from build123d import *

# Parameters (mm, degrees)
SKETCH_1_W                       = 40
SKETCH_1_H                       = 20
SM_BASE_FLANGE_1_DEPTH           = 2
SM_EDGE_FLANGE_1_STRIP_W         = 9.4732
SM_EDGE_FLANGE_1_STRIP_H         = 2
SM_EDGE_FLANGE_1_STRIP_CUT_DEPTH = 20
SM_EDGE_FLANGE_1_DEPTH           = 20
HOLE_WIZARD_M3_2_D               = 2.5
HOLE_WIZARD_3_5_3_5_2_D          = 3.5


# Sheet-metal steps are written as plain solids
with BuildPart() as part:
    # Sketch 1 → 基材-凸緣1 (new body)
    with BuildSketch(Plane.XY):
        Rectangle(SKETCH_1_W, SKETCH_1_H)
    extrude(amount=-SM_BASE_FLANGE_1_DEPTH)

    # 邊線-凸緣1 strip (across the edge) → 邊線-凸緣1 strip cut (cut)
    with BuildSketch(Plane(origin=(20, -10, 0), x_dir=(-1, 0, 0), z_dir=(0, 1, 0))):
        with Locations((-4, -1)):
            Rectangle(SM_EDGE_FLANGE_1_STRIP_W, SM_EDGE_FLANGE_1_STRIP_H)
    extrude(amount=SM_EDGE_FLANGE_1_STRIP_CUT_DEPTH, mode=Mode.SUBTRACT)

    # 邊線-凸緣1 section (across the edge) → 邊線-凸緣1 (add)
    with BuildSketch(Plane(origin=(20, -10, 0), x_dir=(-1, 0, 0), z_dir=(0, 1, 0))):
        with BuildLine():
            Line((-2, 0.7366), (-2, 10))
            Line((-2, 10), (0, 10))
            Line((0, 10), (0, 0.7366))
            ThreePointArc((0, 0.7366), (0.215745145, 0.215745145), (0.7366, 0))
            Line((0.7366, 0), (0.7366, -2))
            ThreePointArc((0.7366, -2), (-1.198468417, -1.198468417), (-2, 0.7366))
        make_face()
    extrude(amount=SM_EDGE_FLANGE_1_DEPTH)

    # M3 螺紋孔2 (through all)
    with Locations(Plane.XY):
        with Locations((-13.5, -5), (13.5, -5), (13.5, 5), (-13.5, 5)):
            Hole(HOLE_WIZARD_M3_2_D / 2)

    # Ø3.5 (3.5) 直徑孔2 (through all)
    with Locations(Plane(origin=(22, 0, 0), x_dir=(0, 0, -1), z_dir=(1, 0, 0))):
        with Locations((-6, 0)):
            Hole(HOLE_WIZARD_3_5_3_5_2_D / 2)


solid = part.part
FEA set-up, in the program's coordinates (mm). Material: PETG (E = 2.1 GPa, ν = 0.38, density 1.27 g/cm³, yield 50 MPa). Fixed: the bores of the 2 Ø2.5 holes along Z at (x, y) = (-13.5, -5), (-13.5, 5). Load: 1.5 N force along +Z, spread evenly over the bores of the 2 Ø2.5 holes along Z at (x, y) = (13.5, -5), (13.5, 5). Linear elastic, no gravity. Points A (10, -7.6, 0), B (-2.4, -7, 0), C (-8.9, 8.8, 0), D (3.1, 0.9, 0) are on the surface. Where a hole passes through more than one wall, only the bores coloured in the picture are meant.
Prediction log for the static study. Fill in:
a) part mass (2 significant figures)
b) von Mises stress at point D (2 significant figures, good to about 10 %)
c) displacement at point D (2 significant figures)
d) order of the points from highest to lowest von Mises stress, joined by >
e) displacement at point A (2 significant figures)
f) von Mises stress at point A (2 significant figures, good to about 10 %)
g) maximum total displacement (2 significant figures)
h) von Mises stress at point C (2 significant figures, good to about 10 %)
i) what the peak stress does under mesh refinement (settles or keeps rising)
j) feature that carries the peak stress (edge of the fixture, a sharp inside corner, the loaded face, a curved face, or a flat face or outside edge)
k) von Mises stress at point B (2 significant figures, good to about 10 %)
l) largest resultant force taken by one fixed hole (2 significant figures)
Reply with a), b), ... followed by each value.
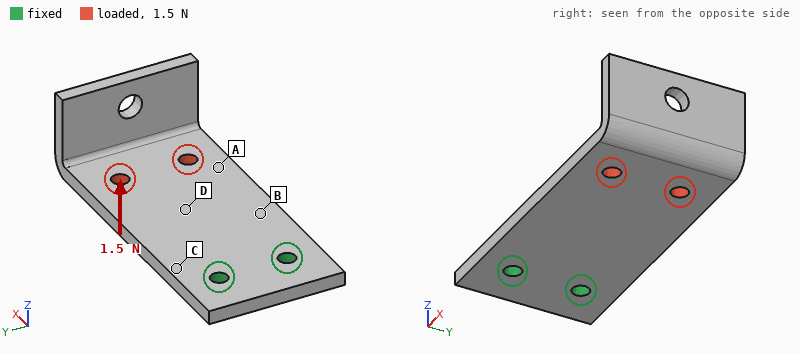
a) 2.5 g
b) 1.1 MPa
c) 0.15 mm
d) C > B > D > A
e) 0.26 mm
f) 0.46 MPa
g) 0.51 mm
h) 2.4 MPa
i) keeps rising
j) edge of the fixture
k) 1.7 MPa
l) 0.75 N
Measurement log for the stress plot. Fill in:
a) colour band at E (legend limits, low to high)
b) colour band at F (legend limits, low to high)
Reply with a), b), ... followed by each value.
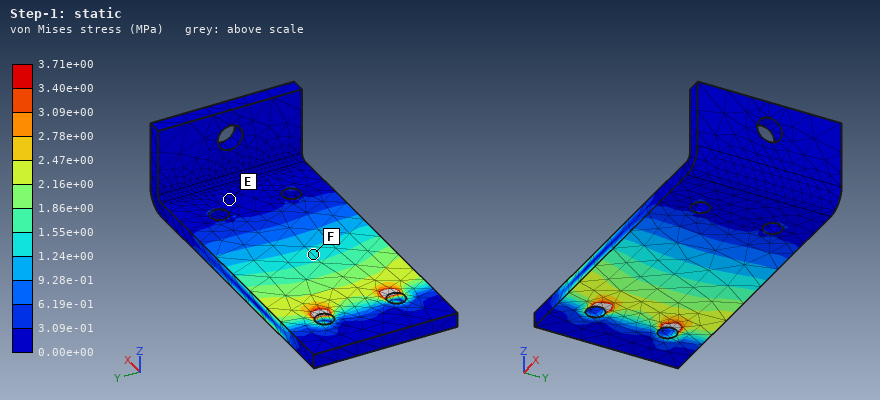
a) 0.00e+00 to 3.09e-01 MPa
b) 1.24e+00 to 1.55e+00 MPa
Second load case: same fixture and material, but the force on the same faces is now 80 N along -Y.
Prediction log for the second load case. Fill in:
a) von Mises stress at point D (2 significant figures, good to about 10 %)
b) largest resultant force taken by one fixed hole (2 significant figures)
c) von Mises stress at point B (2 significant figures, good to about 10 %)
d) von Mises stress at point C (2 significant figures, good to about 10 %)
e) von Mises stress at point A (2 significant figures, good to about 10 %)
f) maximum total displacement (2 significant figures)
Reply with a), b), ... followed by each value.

a) 5.2 MPa
b) 190 N
c) 7.2 MPa
d) 9.8 MPa
e) 2.9 MPa
f) 0.46 mm
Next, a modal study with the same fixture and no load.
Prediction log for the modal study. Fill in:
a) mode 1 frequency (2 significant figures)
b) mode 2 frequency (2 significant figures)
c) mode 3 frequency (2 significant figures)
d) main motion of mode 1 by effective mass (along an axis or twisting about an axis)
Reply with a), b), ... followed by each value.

a) 240 Hz
b) 760 Hz
c) 1300 Hz
d) along Z
